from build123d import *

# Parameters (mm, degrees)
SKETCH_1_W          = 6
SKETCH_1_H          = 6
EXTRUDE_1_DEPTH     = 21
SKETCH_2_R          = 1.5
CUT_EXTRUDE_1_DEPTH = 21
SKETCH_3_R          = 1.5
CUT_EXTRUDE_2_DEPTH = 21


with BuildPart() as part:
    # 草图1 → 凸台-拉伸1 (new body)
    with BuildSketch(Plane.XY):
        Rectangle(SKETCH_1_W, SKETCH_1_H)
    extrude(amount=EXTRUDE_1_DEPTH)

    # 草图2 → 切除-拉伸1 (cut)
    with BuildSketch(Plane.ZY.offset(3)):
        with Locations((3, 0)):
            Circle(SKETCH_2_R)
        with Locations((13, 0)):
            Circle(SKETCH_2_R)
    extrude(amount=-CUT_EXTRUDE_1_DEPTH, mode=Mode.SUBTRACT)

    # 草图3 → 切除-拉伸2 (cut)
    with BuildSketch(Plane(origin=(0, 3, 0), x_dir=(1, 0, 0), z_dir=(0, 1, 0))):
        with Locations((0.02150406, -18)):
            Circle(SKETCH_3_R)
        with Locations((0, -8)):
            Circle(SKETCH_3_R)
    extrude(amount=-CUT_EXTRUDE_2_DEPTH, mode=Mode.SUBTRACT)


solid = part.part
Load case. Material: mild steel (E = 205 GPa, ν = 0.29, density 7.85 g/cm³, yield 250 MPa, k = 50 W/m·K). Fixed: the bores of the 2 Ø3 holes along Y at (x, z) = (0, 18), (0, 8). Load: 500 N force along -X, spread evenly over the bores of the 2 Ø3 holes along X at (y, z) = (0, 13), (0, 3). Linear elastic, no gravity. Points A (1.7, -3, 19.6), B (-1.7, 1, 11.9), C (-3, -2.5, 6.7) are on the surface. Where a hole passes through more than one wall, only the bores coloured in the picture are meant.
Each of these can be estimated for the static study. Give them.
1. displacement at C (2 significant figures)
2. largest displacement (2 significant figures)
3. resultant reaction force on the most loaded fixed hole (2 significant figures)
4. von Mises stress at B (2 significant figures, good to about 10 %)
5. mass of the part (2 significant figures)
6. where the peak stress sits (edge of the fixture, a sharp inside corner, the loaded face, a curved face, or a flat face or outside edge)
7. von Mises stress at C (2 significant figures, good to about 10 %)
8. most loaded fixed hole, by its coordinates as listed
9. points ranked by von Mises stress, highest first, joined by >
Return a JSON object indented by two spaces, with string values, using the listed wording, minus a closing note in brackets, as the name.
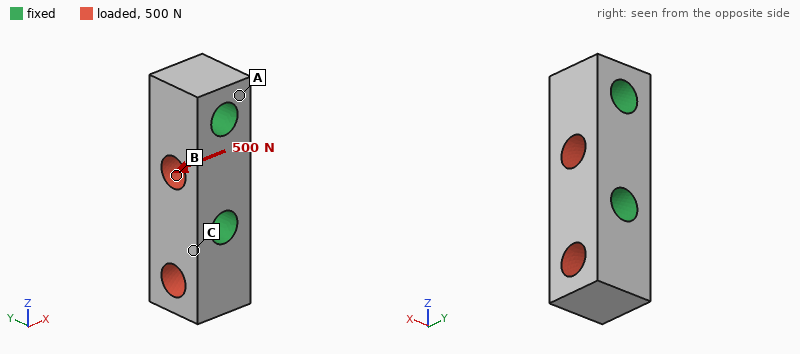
{
  "displacement at C": "0.29 µm",
  "largest displacement": "1.8 µm",
  "resultant reaction force on the most loaded fixed hole": "390 N",
  "von Mises stress at B": "10 MPa",
  "mass of the part": "4.6 g",
  "where the peak stress sits": "edge of the fixture",
  "von Mises stress at C": "25 MPa",
  "most loaded fixed hole, by its coordinates as listed": "(0, 8)",
  "points ranked by von Mises stress, highest first, joined by >": "C > B > A"
}
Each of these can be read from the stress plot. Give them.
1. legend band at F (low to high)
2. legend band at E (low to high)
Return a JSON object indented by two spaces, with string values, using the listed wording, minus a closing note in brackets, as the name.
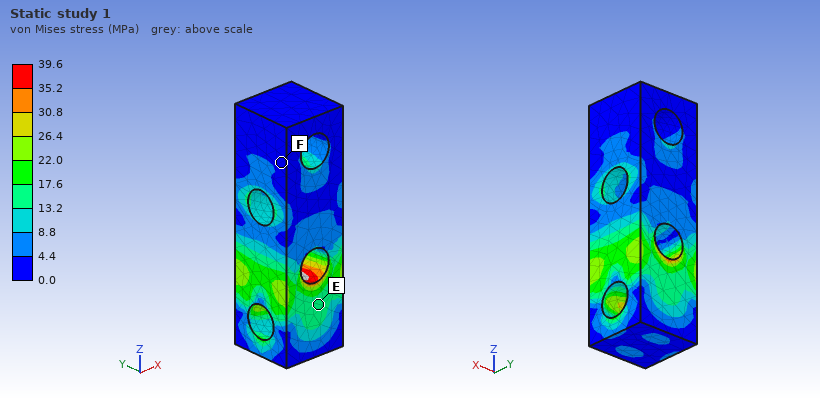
{
  "legend band at F": "0.0 to 4.4 MPa",
  "legend band at E": "13.2 to 17.6 MPa"
}
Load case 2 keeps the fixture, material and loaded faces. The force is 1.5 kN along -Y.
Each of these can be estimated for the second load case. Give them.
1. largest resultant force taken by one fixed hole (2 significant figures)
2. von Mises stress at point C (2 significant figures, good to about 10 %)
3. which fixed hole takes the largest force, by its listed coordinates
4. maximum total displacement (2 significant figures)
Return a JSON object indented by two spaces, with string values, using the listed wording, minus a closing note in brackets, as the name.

{
  "largest resultant force taken by one fixed hole": "1.1 kN",
  "von Mises stress at point C": "35 MPa",
  "which fixed hole takes the largest force, by its listed coordinates": "(0, 8)",
  "maximum total displacement": "5.2 µm"
}
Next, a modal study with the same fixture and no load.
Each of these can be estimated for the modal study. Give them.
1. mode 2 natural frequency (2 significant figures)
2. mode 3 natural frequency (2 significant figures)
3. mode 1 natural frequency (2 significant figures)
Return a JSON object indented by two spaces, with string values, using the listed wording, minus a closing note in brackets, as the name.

{
  "mode 2 natural frequency": "58 kHz",
  "mode 3 natural frequency": "90 kHz",
  "mode 1 natural frequency": "58 kHz"
}
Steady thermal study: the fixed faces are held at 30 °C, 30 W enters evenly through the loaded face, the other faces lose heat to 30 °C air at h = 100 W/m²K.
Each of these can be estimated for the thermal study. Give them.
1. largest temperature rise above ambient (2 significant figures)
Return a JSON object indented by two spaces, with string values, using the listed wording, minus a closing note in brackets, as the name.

{
  "largest temperature rise above ambient": "49 K"
}
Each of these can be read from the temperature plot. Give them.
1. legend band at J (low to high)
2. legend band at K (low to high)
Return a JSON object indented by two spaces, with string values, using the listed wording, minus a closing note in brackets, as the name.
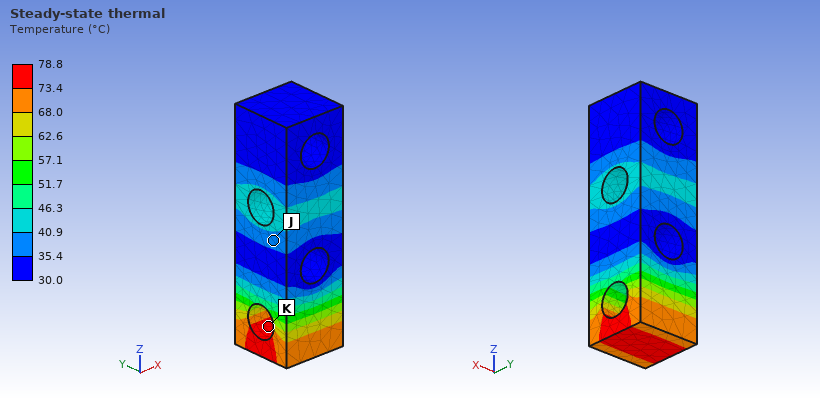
{
  "legend band at J": "35.4 to 40.9 °C",
  "legend band at K": "73.4 to 78.8 °C"
}
